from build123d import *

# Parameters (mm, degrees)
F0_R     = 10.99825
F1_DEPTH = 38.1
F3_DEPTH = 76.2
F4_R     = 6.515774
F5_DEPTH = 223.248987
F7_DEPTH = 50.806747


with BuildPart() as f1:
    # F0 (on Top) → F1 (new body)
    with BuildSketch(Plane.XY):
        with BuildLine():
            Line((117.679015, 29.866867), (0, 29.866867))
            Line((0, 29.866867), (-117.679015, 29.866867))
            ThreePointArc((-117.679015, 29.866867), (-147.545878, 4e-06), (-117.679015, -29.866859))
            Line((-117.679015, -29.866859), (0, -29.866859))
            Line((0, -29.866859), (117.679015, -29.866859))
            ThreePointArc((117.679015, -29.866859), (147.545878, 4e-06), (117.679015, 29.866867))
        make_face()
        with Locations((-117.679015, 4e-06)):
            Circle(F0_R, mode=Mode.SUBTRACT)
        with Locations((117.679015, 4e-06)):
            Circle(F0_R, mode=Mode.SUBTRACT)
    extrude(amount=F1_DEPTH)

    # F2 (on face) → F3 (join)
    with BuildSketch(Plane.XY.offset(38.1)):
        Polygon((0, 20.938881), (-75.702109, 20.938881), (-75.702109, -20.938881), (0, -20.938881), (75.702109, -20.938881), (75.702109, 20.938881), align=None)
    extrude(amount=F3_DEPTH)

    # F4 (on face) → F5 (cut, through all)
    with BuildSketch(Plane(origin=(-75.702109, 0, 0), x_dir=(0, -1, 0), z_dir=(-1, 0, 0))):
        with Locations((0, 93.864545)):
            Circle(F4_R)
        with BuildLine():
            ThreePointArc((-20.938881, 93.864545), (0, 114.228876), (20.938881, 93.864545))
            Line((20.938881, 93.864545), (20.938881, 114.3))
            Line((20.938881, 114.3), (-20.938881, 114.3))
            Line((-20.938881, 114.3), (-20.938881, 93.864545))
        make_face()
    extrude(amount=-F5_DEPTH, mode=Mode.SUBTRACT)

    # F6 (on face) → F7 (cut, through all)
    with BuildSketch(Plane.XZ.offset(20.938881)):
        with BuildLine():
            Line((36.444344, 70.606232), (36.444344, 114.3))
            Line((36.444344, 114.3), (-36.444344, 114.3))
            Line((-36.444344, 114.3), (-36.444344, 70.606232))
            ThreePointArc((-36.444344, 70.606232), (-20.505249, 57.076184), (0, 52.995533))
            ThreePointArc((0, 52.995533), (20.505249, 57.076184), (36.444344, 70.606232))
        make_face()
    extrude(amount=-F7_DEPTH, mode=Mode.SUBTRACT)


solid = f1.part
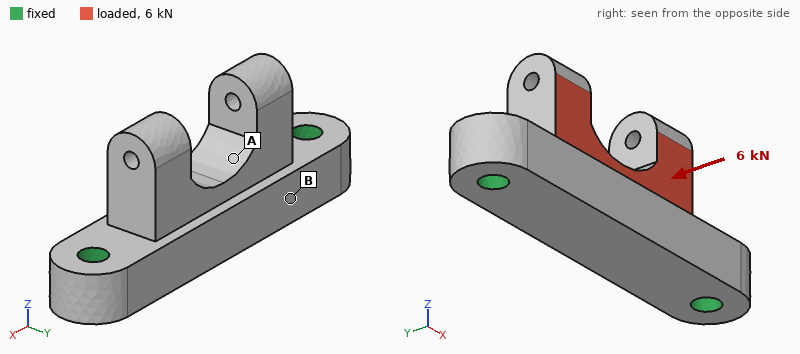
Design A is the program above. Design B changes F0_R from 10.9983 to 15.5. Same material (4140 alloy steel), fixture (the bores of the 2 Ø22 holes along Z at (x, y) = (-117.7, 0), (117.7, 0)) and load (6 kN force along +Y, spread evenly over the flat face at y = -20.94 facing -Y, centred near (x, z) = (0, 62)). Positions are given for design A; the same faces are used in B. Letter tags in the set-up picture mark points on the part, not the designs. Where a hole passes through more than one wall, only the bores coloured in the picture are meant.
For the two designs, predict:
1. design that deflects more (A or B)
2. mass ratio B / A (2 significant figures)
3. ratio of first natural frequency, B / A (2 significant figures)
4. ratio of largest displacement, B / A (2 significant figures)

A
0.97
1.1
0.85
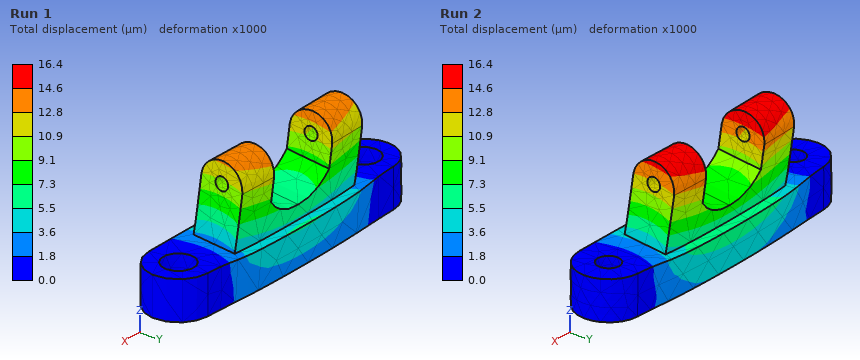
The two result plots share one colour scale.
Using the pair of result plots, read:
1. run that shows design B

Run 1
